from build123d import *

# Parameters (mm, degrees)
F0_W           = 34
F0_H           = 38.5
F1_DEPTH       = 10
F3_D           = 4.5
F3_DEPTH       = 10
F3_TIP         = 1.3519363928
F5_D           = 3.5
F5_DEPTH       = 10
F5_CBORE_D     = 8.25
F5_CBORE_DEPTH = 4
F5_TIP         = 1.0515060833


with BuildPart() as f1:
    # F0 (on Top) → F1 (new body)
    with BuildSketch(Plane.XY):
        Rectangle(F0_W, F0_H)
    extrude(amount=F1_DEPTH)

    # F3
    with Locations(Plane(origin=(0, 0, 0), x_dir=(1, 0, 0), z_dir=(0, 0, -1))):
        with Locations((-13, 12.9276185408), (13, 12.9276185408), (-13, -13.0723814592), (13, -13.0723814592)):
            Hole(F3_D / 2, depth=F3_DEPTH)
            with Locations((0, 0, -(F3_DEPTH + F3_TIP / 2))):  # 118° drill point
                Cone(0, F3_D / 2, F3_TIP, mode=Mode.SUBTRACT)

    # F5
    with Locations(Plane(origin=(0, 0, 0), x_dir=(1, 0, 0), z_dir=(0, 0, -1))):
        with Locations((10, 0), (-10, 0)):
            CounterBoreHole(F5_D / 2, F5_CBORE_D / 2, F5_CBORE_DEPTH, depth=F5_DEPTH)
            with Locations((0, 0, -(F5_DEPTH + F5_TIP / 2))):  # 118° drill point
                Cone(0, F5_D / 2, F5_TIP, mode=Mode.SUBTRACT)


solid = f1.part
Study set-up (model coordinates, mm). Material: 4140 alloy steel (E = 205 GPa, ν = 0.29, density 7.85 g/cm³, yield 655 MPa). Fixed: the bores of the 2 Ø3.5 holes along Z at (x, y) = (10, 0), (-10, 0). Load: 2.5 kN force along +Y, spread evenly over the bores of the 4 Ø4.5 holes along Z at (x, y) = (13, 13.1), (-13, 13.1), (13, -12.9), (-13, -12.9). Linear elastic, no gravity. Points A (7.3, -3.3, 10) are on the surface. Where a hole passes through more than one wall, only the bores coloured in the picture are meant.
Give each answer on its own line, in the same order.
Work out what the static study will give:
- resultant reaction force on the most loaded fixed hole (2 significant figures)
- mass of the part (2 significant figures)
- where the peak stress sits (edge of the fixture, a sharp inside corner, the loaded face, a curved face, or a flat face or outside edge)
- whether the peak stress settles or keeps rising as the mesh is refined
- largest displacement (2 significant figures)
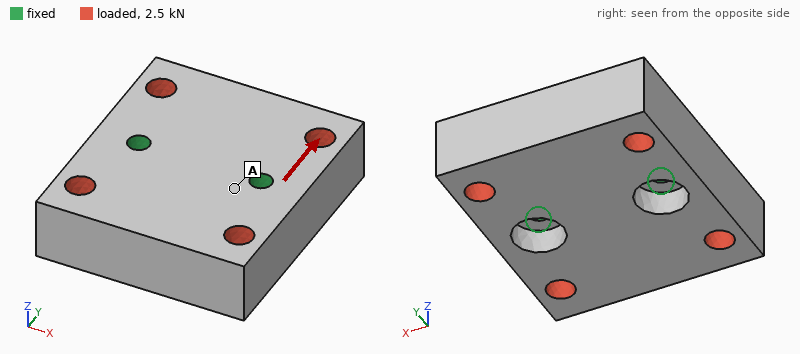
1.3 kN
93 g
edge of the fixture
keeps rising
2.9 µm
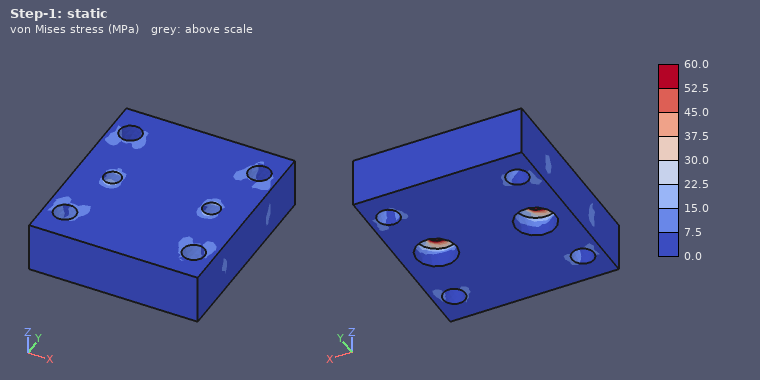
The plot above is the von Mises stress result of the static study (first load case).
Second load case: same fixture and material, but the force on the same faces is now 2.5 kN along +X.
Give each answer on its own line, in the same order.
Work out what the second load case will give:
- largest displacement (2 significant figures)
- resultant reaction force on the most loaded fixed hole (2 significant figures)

1.6 µm
1.3 kN
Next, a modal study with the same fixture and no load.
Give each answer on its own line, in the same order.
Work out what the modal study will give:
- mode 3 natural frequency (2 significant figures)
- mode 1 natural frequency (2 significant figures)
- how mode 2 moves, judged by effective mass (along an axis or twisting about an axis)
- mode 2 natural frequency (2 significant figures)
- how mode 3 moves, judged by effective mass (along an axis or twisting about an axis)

21 kHz
9100 Hz
along Z
17 kHz
twisting about Z
